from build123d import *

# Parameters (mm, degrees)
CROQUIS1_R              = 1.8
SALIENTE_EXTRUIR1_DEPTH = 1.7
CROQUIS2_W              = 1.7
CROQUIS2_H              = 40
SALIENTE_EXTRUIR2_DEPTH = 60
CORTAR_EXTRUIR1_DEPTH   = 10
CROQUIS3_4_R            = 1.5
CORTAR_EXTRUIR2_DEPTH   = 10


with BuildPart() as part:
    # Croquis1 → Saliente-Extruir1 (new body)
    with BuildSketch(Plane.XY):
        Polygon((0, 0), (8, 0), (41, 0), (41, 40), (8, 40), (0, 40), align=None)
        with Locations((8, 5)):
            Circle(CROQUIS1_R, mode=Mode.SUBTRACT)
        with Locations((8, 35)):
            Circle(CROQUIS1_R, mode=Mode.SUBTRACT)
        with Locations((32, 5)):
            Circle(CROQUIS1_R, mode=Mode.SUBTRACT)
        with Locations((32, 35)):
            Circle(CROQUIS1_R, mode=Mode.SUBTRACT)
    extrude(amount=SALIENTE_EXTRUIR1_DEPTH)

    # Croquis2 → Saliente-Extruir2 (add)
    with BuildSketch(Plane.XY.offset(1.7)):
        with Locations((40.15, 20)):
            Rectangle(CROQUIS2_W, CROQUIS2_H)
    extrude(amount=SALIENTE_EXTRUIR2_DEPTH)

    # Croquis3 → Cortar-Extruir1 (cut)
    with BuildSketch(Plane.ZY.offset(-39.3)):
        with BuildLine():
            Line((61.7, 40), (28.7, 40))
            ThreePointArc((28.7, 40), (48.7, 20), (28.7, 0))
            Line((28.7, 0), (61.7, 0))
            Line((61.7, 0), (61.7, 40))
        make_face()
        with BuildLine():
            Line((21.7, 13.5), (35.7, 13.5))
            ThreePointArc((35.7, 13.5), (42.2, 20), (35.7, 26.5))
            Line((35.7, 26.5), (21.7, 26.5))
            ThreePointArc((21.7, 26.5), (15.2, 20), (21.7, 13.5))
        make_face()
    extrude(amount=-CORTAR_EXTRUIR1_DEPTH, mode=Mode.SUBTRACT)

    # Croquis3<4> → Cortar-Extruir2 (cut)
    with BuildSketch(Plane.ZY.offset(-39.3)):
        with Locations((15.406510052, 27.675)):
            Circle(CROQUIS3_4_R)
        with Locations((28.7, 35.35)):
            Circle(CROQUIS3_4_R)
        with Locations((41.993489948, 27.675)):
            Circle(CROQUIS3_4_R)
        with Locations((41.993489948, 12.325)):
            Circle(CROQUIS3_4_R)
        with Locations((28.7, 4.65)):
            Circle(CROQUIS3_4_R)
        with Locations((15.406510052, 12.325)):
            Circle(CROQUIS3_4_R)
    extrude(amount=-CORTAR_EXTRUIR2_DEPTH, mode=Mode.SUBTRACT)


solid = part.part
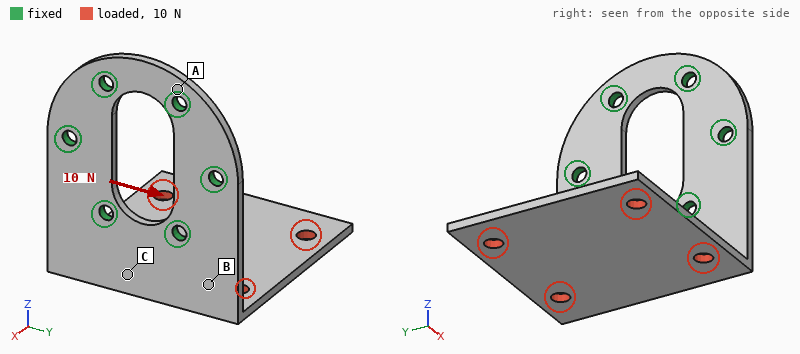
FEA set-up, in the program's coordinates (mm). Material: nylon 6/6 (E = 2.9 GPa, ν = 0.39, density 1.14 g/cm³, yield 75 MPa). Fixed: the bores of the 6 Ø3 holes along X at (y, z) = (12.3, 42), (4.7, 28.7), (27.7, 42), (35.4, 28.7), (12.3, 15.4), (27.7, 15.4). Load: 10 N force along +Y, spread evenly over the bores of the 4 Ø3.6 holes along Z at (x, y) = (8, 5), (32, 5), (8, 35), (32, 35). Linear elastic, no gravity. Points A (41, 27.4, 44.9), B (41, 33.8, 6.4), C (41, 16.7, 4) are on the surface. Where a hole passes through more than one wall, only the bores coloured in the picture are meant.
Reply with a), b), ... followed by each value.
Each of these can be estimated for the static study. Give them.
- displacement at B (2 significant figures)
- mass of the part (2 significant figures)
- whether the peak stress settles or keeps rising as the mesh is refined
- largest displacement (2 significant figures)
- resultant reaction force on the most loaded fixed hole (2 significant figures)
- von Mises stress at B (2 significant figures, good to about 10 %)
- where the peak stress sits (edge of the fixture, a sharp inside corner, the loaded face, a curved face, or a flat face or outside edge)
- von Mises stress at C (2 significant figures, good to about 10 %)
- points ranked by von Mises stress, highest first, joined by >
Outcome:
a) 0.14 mm
b) 5.7 g
c) keeps rising
d) 0.76 mm
e) 12 N
f) 1.9 MPa
g) edge of the fixture
h) 3.9 MPa
i) C > B > A
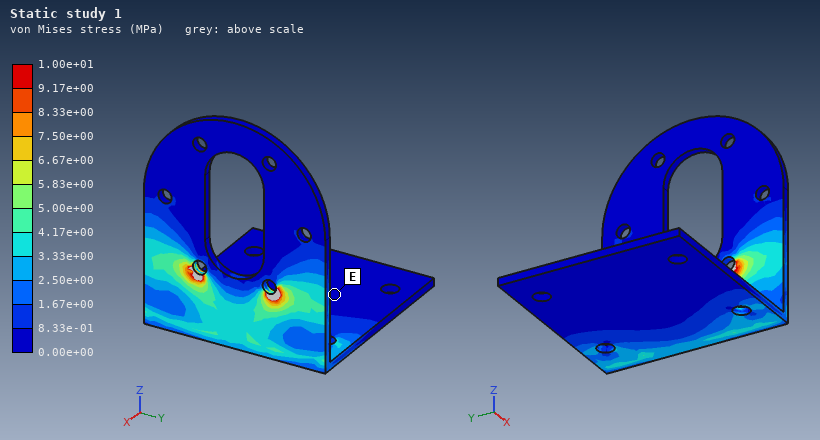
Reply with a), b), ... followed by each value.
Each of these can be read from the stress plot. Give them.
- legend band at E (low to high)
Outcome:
a) 0.00e+00 to 8.33e-01 MPa
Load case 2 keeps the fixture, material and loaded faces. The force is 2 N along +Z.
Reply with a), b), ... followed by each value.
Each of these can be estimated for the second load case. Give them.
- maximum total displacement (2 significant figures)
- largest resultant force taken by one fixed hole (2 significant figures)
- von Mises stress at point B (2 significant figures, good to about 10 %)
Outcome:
a) 0.76 mm
b) 1.00 N
c) 1.7 MPa
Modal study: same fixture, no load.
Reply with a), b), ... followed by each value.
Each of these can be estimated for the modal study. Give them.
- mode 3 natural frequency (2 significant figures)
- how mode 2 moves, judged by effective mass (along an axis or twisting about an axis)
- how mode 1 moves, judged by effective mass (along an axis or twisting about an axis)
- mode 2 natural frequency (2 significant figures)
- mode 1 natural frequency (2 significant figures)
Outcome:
a) 640 Hz
b) along Y
c) along Z
d) 380 Hz
e) 180 Hz
